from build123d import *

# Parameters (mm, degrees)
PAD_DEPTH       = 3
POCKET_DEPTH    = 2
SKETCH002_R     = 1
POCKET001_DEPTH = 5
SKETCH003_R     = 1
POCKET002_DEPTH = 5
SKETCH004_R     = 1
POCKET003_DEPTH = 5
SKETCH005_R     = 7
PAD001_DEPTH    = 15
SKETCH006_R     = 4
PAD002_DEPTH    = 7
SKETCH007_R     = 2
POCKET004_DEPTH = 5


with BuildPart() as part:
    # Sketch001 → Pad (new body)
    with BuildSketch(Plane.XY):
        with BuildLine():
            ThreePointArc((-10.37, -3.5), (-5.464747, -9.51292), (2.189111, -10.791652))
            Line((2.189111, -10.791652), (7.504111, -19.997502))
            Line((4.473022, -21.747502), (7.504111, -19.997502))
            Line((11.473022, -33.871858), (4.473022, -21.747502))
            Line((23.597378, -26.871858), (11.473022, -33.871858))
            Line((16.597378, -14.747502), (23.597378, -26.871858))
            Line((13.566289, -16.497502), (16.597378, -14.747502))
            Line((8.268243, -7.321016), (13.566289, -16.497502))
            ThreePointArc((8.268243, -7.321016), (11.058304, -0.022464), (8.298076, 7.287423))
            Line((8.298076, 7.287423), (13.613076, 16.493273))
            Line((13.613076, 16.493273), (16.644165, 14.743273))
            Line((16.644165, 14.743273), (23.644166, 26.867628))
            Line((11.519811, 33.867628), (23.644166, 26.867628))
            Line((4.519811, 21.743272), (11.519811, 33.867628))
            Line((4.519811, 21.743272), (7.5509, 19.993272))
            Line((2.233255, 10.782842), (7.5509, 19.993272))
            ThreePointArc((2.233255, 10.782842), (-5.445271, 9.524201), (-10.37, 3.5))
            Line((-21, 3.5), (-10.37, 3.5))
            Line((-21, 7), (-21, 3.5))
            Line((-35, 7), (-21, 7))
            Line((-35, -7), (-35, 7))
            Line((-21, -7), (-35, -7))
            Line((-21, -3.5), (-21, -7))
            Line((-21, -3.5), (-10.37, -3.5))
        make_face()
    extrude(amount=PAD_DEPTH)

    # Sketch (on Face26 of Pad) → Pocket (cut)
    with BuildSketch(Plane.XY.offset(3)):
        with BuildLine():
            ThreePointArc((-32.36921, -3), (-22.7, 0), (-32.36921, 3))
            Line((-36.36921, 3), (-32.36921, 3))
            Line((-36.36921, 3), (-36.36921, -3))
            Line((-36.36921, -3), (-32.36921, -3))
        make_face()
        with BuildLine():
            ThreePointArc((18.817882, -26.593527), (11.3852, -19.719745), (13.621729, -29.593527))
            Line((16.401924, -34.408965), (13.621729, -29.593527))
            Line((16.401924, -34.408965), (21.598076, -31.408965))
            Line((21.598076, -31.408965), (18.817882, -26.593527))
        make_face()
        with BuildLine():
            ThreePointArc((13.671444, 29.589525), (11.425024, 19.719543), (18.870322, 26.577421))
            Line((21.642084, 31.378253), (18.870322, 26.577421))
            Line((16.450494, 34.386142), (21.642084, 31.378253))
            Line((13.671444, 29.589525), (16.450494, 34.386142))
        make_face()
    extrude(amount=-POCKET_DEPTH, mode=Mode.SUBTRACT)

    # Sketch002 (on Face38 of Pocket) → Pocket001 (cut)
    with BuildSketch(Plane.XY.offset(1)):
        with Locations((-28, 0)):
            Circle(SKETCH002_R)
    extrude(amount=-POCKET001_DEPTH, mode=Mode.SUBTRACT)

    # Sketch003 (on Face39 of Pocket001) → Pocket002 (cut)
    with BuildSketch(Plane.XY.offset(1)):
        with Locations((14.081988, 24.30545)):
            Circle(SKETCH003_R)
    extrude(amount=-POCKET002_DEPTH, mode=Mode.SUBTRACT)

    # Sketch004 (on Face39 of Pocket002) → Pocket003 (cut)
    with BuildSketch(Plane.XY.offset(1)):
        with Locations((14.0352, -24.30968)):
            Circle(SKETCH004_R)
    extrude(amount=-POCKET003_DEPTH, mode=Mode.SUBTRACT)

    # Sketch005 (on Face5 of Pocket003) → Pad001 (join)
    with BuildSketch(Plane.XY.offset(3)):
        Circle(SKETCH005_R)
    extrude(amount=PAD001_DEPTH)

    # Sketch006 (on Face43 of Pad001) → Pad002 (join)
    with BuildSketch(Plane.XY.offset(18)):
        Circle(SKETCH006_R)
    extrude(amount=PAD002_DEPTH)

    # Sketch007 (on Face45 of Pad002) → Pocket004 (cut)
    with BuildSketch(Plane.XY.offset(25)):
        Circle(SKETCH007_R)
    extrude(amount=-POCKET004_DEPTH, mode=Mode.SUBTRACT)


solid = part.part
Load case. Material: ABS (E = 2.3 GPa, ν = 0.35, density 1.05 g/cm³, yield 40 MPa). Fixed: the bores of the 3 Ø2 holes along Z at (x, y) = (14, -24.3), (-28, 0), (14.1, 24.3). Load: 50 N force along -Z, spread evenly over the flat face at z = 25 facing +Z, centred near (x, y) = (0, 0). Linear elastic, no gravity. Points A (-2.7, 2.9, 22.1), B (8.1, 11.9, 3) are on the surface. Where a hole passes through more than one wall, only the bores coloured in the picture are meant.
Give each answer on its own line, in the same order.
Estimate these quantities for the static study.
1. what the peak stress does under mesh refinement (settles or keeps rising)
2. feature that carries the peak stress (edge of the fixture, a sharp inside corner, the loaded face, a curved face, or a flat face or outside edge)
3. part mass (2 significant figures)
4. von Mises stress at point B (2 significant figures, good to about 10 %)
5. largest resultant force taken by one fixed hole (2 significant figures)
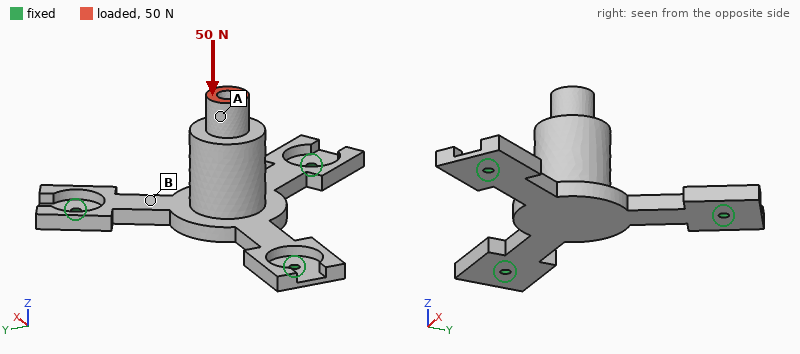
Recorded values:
keeps rising
edge of the fixture
5.8 g
11 MPa
61 N
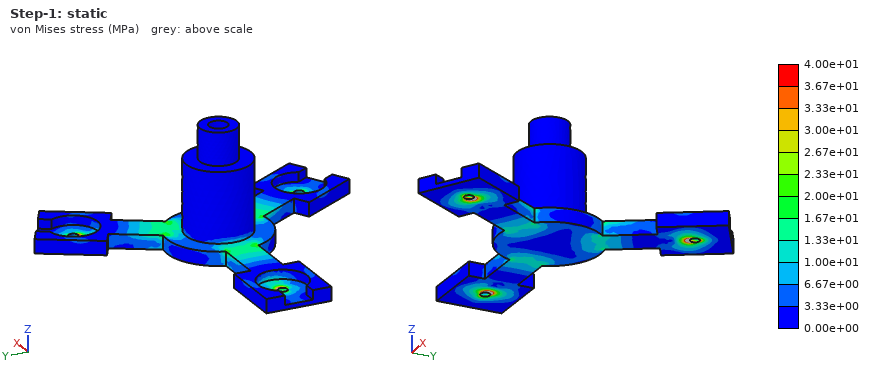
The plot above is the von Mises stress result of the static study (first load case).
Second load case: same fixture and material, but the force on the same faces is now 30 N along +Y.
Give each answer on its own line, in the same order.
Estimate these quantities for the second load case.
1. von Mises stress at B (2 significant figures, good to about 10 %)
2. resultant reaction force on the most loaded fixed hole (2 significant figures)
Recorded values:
14 MPa
26 N
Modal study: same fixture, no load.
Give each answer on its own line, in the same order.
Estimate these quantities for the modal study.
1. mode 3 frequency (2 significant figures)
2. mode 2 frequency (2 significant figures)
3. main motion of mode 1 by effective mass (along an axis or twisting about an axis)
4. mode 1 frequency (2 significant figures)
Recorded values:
990 Hz
990 Hz
along Z
660 Hz
